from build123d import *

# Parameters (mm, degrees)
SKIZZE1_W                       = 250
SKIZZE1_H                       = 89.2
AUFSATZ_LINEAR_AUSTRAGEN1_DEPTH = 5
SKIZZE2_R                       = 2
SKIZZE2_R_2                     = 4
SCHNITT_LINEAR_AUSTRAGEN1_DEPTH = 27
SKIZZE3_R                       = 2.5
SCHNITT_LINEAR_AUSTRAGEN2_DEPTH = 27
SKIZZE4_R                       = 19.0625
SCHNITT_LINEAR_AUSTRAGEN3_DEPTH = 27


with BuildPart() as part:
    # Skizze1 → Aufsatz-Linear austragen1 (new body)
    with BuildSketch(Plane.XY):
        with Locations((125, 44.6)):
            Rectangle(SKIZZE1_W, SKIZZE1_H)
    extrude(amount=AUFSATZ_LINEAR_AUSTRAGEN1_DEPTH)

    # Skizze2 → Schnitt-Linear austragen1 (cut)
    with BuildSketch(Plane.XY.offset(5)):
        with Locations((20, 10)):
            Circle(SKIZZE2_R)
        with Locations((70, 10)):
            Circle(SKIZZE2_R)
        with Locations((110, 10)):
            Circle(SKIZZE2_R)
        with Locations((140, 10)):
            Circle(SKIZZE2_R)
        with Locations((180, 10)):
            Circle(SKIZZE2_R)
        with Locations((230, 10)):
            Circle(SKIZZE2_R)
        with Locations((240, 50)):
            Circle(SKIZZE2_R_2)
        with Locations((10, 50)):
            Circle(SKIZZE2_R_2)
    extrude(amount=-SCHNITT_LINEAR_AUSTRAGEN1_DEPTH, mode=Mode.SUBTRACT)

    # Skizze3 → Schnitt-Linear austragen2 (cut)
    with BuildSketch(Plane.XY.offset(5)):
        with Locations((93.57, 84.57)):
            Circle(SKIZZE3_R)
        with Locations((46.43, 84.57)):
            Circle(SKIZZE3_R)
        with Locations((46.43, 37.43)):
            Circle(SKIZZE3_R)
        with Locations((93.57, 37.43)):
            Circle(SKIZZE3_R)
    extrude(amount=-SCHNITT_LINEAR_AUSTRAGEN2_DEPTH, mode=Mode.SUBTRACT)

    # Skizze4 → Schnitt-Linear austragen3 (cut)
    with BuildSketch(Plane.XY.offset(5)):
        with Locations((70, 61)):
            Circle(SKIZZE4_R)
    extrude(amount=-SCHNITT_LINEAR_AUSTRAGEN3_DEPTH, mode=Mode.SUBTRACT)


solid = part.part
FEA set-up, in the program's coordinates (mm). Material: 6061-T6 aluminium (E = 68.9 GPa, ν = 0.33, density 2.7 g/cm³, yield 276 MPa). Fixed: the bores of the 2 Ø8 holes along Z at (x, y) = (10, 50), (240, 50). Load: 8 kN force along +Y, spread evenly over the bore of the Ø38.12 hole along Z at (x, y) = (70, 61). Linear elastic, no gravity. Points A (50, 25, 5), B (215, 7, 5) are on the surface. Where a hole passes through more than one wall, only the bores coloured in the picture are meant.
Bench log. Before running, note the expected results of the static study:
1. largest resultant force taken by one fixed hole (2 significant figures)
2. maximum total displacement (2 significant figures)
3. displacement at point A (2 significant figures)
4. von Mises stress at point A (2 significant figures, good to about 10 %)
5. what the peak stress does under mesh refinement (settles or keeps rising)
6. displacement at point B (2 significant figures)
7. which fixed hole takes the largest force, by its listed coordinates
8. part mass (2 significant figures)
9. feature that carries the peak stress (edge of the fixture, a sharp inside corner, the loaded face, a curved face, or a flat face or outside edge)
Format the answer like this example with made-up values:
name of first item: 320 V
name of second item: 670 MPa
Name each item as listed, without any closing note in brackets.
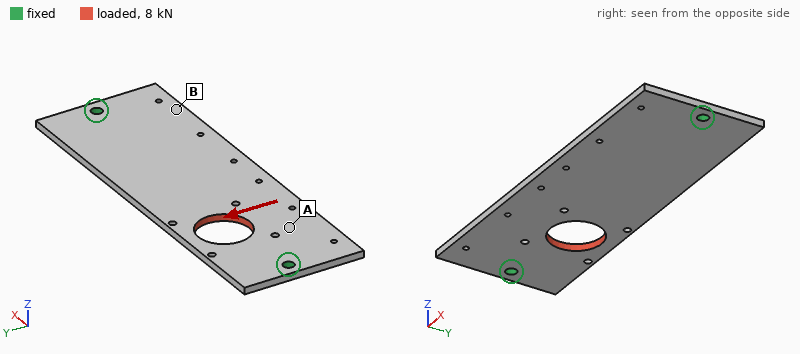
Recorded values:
largest resultant force taken by one fixed hole: 6.1 kN
maximum total displacement: 0.12 mm
displacement at point A: 0.069 mm
von Mises stress at point A: 30 MPa
what the peak stress does under mesh refinement: keeps rising
displacement at point B: 0.042 mm
which fixed hole takes the largest force, by its listed coordinates: (10, 50)
part mass: 280 g
feature that carries the peak stress: edge of the fixture
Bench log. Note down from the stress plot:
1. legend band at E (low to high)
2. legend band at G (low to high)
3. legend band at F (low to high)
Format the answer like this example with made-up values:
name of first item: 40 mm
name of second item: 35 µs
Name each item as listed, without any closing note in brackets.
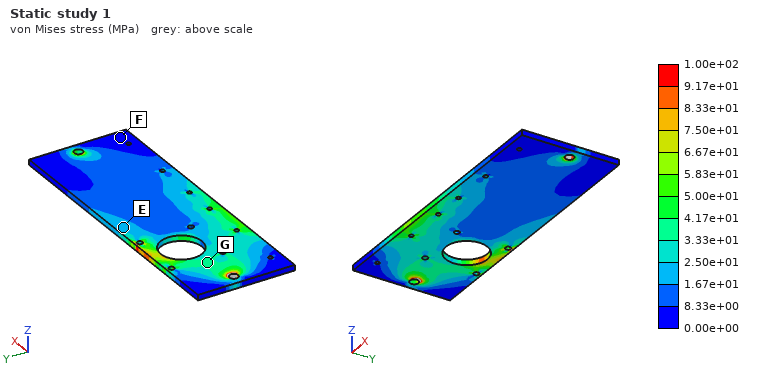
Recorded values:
legend band at E: 1.67e+01 to 2.50e+01 MPa
legend band at G: 3.33e+01 to 4.17e+01 MPa
legend band at F: 0.00e+00 to 8.33e+00 MPa
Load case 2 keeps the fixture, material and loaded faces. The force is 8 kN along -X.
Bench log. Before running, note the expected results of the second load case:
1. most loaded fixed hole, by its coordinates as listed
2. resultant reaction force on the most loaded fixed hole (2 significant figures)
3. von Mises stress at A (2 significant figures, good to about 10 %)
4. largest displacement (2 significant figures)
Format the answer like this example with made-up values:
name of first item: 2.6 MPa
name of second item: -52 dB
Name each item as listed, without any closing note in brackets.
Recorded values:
most loaded fixed hole, by its coordinates as listed: (10, 50)
resultant reaction force on the most loaded fixed hole: 5.0 kN
von Mises stress at A: 9.3 MPa
largest displacement: 34 µm
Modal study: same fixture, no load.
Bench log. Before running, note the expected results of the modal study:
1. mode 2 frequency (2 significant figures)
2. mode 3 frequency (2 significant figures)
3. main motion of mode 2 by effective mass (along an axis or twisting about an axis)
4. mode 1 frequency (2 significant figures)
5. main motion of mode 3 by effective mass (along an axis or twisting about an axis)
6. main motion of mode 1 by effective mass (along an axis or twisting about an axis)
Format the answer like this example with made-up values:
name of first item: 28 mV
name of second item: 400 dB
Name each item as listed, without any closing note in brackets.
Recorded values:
mode 2 frequency: 660 Hz
mode 3 frequency: 1100 Hz
main motion of mode 2 by effective mass: twisting about X
mode 1 frequency: 440 Hz
main motion of mode 3 by effective mass: twisting about Y
main motion of mode 1 by effective mass: along Z
